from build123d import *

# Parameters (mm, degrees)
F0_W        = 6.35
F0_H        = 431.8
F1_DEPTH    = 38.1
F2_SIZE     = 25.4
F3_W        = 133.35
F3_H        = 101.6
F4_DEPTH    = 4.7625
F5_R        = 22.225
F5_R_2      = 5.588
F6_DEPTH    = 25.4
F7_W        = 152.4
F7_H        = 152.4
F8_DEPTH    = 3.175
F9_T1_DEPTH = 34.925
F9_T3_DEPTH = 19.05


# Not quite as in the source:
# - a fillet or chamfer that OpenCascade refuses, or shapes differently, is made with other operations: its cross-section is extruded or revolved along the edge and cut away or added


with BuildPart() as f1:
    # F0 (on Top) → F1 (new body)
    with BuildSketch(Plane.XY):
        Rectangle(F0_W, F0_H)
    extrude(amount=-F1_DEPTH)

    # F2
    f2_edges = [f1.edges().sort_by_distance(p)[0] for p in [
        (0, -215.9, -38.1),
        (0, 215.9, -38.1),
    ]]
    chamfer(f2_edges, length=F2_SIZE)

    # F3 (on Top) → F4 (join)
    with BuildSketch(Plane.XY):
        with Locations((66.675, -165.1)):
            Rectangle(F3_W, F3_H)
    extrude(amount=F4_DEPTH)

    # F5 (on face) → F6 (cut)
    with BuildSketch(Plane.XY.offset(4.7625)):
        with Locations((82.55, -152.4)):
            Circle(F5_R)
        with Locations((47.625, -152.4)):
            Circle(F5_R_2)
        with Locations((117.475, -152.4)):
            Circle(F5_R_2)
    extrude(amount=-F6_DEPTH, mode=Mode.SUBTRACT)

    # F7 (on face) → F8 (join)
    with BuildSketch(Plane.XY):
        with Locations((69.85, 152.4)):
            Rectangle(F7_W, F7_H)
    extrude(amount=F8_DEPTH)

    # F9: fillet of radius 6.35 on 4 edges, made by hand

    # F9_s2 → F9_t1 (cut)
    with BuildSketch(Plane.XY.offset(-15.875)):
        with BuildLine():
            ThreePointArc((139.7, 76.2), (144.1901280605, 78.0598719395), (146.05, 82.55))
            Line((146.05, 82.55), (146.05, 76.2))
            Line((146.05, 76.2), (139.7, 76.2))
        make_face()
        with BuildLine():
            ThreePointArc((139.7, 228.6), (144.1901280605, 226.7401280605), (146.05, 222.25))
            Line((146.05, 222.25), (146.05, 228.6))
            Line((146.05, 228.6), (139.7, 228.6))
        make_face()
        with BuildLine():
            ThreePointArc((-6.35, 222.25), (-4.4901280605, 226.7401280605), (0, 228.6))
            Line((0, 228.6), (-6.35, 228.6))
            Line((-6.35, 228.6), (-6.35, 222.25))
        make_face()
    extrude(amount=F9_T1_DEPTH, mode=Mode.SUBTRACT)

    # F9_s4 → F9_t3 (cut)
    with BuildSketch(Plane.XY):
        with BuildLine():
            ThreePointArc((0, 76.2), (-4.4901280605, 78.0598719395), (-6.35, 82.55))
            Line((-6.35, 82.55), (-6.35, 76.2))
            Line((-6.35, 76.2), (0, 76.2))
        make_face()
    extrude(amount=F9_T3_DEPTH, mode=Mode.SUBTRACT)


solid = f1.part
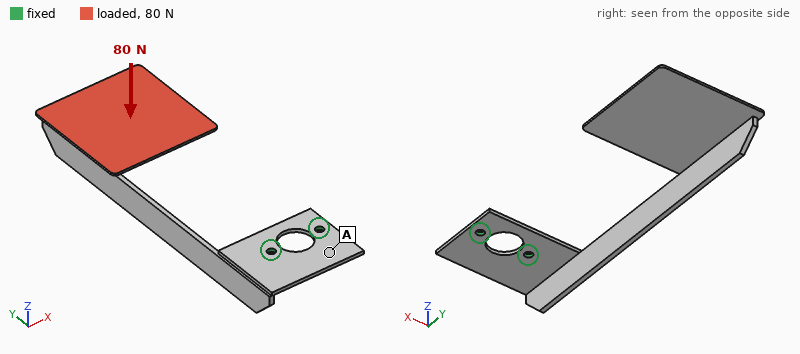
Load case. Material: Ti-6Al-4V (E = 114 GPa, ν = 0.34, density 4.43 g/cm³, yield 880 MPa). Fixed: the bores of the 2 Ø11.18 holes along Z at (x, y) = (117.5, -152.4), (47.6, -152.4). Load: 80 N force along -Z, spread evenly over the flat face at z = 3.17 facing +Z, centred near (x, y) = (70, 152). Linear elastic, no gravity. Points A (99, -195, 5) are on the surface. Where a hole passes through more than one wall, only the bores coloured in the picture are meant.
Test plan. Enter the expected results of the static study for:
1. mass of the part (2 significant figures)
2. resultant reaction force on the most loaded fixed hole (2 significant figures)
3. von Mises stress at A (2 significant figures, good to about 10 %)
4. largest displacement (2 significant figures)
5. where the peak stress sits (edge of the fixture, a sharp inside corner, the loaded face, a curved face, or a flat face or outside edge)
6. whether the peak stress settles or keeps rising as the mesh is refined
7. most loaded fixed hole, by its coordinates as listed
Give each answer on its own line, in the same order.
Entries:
1.0 kg
71 N
13 MPa
5.1 mm
edge of the fixture
keeps rising
(47.6, -152.4)
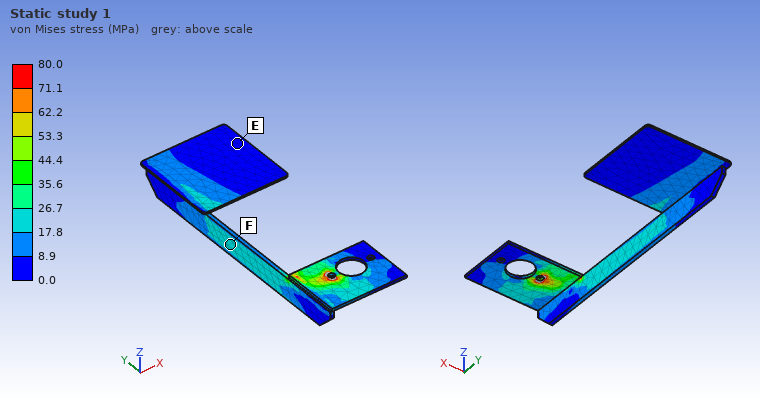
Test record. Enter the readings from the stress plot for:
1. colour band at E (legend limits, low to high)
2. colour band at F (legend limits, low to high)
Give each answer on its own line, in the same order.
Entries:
0.0 to 8.9 MPa
17.8 to 26.7 MPa
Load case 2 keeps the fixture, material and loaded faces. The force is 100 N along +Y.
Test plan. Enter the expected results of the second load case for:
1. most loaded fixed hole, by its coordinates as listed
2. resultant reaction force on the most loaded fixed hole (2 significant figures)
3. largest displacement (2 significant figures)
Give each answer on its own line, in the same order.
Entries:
(47.6, -152.4)
78 N
4.9 mm
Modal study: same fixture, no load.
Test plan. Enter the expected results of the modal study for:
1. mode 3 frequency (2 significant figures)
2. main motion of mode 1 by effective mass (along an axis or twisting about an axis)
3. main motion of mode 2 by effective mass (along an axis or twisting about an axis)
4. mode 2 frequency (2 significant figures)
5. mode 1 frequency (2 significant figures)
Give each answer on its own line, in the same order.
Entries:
84 Hz
along X
along Z
38 Hz
24 Hz
